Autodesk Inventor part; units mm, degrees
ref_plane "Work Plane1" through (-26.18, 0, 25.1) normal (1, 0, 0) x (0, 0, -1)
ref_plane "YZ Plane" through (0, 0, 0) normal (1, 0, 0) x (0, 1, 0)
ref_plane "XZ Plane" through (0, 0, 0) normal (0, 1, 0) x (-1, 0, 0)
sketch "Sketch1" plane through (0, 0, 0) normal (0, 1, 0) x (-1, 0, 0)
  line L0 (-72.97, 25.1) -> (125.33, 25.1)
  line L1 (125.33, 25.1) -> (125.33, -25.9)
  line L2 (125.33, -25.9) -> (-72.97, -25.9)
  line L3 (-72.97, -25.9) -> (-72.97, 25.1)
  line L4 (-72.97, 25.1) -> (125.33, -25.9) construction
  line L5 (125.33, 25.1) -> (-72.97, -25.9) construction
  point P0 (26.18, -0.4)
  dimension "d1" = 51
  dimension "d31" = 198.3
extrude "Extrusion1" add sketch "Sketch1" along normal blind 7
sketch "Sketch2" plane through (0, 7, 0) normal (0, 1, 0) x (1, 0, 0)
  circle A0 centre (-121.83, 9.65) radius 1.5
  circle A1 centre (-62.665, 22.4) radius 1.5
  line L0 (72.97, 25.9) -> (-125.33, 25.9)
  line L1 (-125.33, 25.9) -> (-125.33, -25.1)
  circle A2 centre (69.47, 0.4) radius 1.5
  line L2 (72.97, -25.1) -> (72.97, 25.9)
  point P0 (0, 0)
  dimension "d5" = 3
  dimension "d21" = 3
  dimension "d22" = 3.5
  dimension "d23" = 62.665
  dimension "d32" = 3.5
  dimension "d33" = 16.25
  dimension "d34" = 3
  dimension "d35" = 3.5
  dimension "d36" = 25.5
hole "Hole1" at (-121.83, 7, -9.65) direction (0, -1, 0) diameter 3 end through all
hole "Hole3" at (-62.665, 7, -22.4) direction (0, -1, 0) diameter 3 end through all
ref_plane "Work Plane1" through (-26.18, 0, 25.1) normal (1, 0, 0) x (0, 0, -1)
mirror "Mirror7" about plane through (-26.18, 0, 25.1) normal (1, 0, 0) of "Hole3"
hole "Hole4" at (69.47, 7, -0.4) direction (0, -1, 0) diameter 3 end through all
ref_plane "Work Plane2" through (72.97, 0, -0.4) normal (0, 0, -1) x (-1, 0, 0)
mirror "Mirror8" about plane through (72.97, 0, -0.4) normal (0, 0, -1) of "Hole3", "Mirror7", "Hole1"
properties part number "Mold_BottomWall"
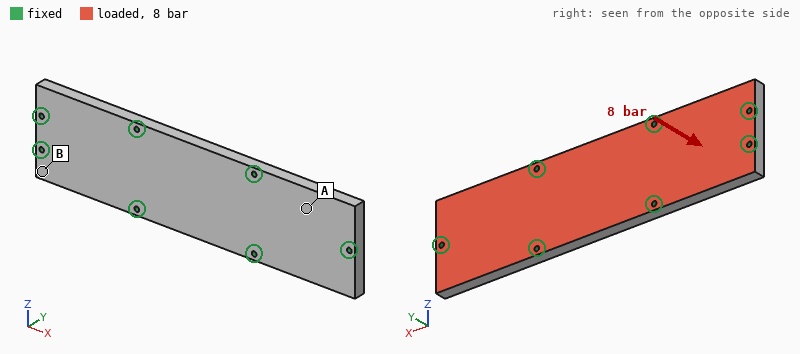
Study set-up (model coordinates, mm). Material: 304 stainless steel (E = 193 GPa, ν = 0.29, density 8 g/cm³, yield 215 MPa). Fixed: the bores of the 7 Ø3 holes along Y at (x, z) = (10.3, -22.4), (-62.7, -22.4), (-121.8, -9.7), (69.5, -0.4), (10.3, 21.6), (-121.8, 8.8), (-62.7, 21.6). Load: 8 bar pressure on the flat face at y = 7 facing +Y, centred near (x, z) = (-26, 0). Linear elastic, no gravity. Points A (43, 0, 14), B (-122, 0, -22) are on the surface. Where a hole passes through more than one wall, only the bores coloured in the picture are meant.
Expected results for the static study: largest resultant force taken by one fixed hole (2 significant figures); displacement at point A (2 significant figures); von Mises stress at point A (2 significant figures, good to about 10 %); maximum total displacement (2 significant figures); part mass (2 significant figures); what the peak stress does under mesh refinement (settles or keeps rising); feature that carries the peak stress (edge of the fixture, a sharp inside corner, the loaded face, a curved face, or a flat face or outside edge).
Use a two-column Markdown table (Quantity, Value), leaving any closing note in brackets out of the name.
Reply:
| Quantity | Value |
|---|---|
| largest resultant force taken by one fixed hole | 1.4 kN |
| displacement at point A | 9.6 µm |
| von Mises stress at point A | 19 MPa |
| maximum total displacement | 15 µm |
| part mass | 560 g |
| what the peak stress does under mesh refinement | keeps rising |
| feature that carries the peak stress | edge of the fixture |
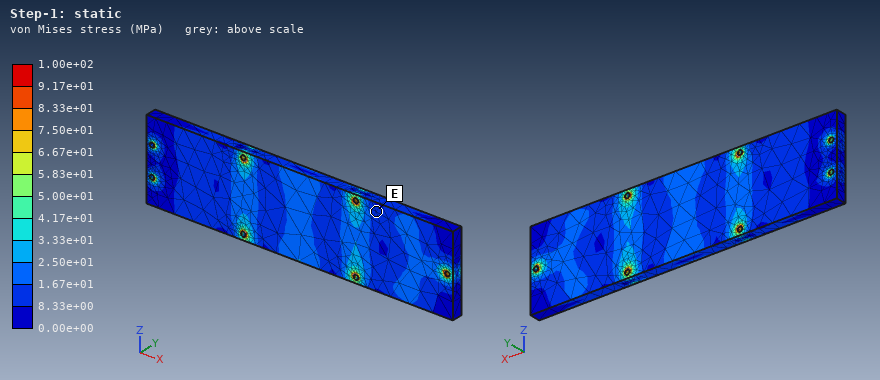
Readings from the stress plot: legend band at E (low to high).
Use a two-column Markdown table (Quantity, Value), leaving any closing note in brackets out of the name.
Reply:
| Quantity | Value |
|---|---|
| legend band at E | 8.33e+00 to 1.67e+01 MPa |
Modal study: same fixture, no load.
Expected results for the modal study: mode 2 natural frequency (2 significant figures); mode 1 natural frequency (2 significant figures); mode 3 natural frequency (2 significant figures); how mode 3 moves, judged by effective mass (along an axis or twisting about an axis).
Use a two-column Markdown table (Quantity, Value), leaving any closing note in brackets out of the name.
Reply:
| Quantity | Value |
|---|---|
| mode 2 natural frequency | 6100 Hz |
| mode 1 natural frequency | 5100 Hz |
| mode 3 natural frequency | 6400 Hz |
| how mode 3 moves, judged by effective mass | along Y |
